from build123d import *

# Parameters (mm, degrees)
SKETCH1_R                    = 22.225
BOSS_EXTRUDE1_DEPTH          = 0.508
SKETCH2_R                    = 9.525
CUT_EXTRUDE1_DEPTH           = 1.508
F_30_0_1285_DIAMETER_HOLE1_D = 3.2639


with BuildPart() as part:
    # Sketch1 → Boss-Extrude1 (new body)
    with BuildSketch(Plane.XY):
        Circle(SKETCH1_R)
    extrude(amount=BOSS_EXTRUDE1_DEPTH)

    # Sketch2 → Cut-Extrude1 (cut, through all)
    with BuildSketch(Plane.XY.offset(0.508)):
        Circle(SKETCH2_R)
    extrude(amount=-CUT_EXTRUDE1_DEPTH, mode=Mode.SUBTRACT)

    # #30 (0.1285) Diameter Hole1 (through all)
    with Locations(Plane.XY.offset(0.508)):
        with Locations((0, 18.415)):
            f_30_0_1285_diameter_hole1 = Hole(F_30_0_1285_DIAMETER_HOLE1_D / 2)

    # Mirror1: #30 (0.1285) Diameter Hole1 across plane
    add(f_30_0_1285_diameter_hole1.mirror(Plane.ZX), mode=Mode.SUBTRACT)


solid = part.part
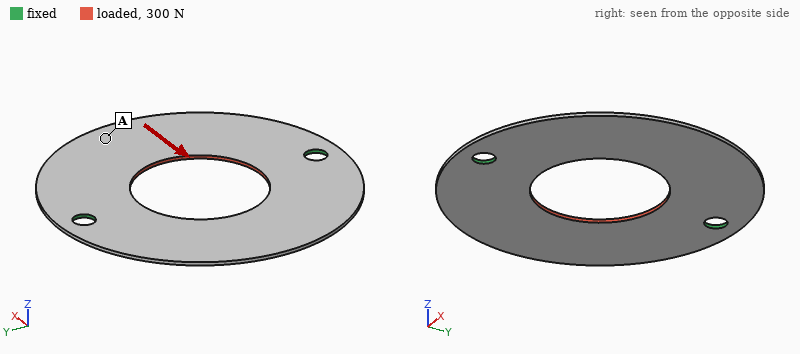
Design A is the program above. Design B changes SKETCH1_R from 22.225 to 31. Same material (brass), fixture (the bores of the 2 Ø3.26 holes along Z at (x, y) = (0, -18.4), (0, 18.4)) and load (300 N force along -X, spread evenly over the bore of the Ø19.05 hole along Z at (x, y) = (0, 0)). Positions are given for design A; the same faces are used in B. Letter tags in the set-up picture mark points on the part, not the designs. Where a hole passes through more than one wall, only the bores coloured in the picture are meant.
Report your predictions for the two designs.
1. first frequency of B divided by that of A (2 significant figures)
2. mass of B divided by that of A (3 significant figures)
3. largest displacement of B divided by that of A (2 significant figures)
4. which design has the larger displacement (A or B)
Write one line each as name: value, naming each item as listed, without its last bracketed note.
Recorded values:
first frequency of B divided by that of A: 0.61
mass of B divided by that of A: 2.17
largest displacement of B divided by that of A: 0.77
which design has the larger displacement: A
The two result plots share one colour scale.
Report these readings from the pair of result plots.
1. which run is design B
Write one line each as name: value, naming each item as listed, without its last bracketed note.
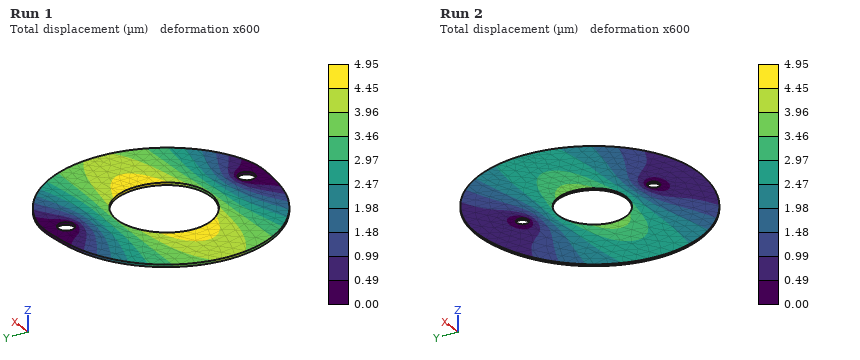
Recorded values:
which run is design B: Run 2
